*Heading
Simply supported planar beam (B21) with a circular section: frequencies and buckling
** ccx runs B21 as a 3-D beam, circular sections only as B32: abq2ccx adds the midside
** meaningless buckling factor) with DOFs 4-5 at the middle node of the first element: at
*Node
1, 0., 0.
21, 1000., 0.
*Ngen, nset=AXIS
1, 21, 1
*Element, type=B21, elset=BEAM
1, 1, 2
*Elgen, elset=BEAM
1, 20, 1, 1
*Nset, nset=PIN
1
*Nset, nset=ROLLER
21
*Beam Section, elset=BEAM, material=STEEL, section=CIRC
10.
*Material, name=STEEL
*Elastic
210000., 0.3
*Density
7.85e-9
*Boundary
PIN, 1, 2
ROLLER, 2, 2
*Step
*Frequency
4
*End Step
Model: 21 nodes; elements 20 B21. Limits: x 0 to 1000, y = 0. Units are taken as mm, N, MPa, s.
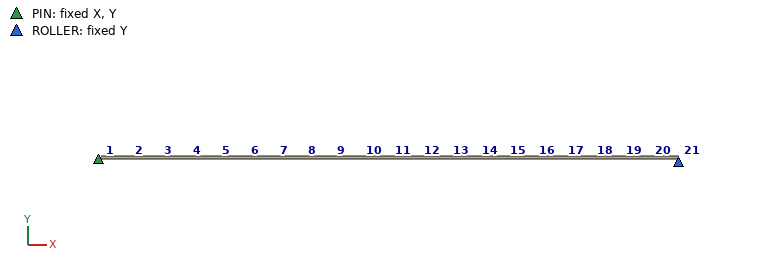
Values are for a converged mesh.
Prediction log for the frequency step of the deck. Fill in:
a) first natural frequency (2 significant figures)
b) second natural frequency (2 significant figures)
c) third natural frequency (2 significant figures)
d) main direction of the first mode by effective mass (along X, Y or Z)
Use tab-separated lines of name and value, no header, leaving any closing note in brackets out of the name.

first natural frequency	20 Hz
second natural frequency	81 Hz
third natural frequency	180 Hz
main direction of the first mode by effective mass	along Y
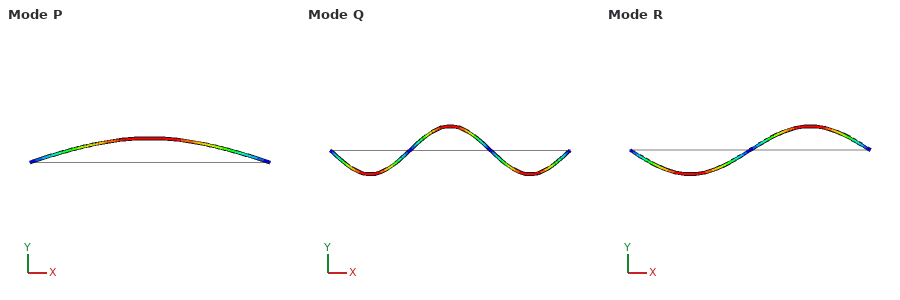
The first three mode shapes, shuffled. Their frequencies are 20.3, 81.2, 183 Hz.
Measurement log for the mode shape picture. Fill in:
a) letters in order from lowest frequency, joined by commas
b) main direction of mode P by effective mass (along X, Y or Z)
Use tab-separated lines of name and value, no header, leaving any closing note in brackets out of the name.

letters in order from lowest frequency, joined by commas	P, R, Q
main direction of mode P by effective mass	along Y
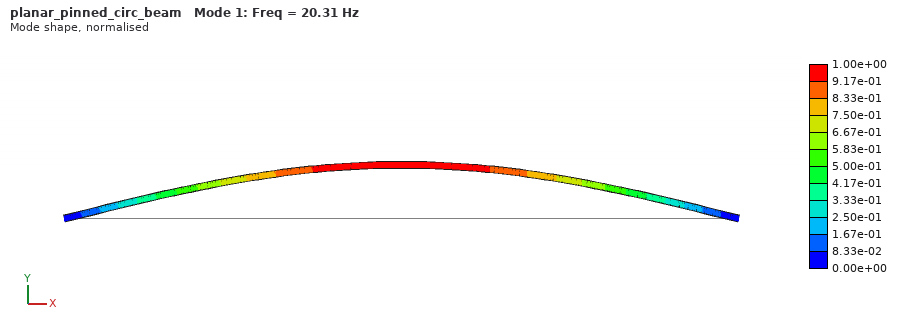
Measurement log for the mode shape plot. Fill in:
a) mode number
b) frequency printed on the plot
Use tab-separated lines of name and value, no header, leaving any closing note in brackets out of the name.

mode number	1
frequency printed on the plot	20.31 Hz
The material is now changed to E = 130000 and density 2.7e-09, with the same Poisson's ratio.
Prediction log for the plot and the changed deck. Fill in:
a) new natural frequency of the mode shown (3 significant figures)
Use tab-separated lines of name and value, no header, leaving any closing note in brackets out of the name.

new natural frequency of the mode shown	27.2 Hz
